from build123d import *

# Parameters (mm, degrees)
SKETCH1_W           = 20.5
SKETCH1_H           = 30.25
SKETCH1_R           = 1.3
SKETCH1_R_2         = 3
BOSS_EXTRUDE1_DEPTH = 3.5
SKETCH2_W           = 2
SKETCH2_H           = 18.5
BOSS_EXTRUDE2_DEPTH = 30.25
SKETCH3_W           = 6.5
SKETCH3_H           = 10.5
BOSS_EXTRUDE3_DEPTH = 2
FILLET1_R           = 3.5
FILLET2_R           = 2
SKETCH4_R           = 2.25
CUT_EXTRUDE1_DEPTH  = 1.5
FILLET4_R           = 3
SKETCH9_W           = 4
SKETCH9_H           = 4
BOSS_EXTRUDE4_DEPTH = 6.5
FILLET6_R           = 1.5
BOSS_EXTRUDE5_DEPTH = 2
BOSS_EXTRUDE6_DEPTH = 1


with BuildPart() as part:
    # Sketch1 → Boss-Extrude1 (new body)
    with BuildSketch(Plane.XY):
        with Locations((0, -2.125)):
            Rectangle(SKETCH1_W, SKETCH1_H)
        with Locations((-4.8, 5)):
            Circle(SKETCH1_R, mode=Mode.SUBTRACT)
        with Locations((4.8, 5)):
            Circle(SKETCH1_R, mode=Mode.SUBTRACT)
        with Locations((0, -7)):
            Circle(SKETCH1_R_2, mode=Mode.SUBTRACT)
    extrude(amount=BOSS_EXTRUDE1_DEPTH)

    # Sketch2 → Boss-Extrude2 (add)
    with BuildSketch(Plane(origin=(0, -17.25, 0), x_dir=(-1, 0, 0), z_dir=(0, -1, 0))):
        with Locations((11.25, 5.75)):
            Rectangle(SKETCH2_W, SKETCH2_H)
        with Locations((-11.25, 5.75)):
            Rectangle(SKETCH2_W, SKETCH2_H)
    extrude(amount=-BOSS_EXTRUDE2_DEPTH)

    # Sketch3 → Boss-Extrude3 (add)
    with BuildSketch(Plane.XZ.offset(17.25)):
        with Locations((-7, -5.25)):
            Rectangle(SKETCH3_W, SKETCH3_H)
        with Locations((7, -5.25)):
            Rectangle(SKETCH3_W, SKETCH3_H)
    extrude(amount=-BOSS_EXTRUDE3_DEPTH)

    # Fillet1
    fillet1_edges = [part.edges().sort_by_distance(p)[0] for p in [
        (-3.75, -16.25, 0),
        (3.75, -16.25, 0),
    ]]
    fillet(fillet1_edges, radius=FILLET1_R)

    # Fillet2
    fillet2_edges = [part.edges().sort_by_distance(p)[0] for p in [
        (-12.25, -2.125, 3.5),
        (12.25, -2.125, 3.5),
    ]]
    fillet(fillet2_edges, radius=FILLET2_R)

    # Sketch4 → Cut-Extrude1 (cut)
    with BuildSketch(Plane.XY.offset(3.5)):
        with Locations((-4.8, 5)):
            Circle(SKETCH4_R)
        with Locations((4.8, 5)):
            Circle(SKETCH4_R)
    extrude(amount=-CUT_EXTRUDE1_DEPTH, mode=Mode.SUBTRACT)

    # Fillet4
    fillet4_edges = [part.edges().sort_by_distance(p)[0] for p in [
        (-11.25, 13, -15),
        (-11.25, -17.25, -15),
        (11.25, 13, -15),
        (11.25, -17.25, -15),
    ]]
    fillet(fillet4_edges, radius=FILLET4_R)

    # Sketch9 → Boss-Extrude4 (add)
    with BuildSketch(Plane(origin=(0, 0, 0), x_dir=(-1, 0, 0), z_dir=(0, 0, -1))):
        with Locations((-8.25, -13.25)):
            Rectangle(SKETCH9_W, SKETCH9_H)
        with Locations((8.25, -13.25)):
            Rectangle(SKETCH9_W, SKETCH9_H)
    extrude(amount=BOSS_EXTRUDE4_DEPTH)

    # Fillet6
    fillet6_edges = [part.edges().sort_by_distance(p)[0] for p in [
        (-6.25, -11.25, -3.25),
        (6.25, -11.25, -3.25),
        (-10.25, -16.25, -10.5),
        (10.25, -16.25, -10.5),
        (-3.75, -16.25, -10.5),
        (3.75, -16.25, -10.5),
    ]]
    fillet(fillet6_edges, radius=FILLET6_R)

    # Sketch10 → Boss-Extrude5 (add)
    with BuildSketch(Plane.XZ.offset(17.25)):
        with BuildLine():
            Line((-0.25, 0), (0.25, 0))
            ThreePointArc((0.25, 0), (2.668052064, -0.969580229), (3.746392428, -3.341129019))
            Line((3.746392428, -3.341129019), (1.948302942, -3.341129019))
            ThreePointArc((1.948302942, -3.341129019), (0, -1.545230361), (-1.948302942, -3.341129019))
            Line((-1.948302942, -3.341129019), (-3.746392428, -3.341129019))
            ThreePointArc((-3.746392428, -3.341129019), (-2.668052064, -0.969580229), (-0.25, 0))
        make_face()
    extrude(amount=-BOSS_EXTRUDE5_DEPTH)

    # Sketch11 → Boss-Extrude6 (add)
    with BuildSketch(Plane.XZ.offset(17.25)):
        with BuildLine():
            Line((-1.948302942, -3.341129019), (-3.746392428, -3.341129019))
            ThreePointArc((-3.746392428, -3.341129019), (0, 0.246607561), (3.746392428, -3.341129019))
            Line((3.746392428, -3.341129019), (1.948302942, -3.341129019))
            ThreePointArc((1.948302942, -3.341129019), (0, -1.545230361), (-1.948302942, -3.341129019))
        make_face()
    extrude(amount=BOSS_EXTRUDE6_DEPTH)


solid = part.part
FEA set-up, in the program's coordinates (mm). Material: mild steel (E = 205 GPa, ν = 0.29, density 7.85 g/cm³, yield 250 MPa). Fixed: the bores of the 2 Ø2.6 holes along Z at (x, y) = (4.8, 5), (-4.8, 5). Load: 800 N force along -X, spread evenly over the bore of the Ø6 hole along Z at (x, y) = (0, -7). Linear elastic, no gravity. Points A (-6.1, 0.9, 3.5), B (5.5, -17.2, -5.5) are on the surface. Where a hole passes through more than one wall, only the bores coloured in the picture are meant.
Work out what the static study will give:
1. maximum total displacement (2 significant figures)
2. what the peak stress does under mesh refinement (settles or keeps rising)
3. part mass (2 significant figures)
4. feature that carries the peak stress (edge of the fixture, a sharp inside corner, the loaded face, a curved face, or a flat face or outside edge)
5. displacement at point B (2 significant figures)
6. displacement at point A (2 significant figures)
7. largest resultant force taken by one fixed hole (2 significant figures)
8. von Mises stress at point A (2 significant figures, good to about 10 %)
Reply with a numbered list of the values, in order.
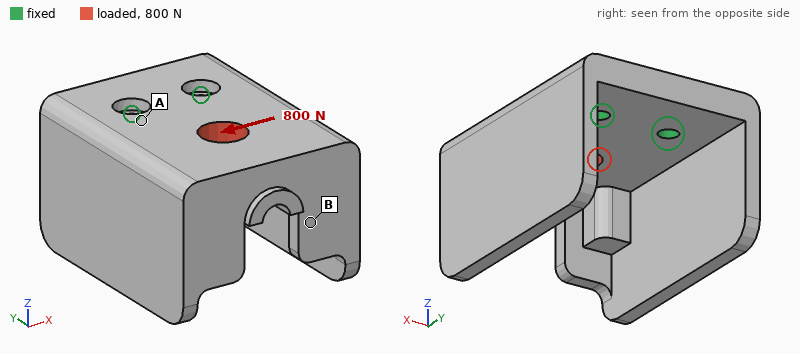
1. 8.1 µm
2. keeps rising
3. 37 g
4. edge of the fixture
5. 7.4 µm
6. 1.7 µm
7. 930 N
8. 18 MPa
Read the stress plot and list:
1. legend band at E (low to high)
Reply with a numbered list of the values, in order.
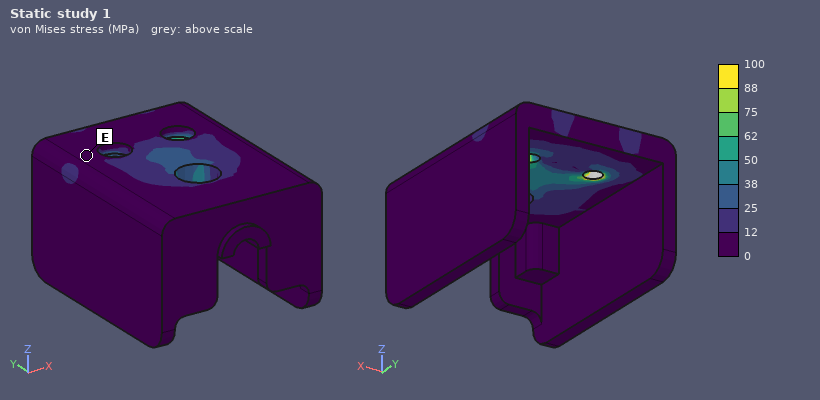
1. 0 to 12 MPa
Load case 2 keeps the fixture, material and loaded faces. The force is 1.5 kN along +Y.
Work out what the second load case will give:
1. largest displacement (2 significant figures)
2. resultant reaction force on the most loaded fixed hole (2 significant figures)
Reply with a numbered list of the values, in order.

1. 8.9 µm
2. 760 N
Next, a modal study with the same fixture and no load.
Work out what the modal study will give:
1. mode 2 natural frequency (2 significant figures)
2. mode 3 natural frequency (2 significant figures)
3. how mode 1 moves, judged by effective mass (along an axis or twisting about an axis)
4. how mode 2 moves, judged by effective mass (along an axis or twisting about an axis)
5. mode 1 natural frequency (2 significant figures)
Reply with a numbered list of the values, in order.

1. 4400 Hz
2. 6600 Hz
3. along Z
4. along X
5. 3100 Hz
